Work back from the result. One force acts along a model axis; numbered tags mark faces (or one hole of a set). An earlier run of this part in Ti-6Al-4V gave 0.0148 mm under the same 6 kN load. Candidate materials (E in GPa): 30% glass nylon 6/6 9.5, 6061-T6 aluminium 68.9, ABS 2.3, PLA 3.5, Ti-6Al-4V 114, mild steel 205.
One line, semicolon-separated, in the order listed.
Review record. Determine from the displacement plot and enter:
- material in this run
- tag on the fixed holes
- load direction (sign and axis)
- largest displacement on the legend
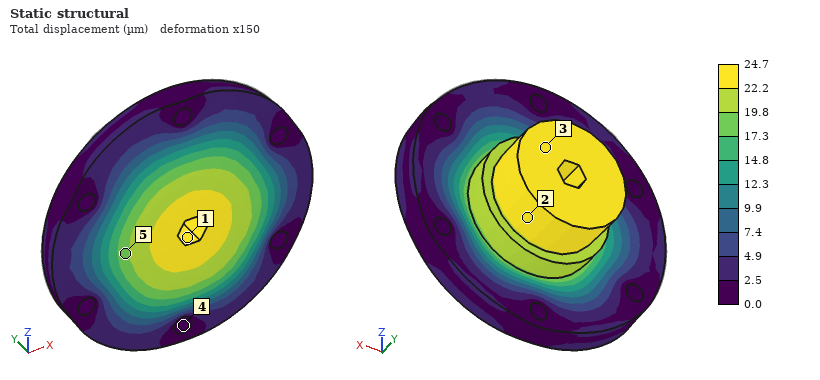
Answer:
6061-T6 aluminium; 4; -Y; 24.7 µm
